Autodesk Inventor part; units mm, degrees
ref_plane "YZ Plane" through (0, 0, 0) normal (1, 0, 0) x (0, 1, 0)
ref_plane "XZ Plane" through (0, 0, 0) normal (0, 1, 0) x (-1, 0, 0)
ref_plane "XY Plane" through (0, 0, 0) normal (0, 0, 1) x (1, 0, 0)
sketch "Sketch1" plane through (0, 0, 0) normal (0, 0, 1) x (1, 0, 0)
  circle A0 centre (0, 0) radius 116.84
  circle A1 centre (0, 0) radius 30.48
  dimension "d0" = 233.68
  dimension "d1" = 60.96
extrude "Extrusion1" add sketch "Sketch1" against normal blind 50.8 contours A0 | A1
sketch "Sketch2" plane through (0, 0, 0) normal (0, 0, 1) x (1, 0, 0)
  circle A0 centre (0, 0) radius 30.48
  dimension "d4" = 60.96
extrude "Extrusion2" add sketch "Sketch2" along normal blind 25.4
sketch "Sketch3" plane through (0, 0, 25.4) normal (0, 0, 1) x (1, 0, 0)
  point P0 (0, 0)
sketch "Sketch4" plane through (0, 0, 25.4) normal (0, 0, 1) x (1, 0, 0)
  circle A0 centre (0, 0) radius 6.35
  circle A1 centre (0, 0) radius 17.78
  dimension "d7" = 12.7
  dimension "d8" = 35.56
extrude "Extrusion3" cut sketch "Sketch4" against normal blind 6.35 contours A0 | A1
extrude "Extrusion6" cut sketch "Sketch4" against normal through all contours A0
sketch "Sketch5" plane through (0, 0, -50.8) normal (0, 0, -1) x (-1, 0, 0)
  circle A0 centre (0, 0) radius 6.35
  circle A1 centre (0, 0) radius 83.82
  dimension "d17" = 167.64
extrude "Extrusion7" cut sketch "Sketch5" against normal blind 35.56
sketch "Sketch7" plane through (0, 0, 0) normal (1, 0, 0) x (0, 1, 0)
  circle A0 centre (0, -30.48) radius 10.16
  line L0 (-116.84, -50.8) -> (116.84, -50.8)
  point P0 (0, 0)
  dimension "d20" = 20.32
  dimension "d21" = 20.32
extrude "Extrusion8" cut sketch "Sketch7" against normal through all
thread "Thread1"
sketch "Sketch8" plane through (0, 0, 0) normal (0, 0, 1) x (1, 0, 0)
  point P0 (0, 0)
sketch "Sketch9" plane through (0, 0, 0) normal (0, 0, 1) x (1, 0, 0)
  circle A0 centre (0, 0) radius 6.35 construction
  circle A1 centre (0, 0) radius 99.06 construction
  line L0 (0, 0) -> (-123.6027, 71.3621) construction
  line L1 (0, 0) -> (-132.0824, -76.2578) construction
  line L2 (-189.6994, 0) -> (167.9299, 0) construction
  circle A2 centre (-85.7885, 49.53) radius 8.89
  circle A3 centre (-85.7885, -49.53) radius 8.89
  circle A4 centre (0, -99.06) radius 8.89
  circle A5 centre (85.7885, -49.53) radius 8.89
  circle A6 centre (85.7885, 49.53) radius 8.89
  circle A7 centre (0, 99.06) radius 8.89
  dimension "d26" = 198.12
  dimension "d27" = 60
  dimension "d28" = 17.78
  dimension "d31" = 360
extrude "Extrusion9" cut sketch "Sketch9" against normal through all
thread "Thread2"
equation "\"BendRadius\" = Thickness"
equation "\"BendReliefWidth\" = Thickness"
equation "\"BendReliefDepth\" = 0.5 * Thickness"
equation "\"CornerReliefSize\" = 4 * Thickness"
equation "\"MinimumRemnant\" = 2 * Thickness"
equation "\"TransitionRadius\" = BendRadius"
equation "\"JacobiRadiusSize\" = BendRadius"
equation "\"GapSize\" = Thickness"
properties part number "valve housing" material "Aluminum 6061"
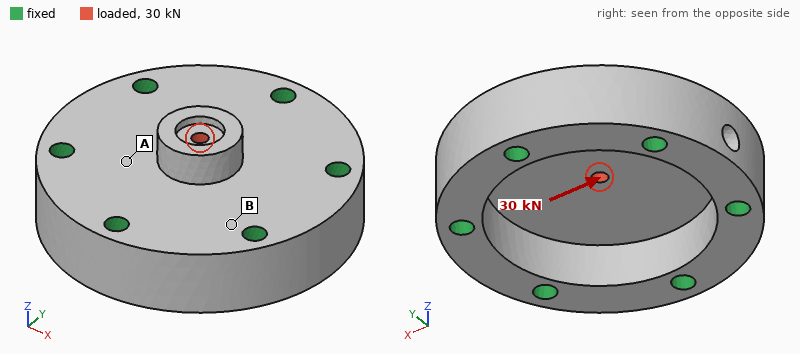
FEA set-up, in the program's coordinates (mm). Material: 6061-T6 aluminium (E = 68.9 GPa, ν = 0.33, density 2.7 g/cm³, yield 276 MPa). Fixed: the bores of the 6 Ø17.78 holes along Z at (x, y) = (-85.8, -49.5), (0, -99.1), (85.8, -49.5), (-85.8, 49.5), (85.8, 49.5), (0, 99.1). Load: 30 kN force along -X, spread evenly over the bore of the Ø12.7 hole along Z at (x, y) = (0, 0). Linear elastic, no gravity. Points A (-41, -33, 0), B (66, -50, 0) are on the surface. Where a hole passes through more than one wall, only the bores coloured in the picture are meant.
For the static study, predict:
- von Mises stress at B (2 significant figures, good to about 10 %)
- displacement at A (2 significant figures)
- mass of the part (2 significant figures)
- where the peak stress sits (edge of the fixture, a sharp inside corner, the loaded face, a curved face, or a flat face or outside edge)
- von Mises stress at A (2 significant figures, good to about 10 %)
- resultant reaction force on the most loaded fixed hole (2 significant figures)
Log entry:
5.2 MPa
7.6 µm
3.7 kg
the loaded face
12 MPa
6.9 kN
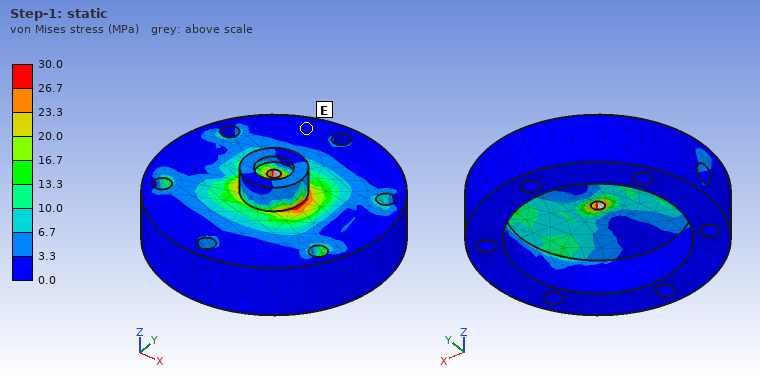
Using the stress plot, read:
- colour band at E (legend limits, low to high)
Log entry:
0.0 to 3.3 MPa
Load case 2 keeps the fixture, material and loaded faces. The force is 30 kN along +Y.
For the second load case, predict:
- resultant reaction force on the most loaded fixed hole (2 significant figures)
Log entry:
7.8 kN
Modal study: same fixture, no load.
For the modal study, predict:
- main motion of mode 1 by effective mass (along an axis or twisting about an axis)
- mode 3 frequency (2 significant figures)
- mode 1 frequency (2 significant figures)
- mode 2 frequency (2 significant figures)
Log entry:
along Z
6800 Hz
3800 Hz
6800 Hz
